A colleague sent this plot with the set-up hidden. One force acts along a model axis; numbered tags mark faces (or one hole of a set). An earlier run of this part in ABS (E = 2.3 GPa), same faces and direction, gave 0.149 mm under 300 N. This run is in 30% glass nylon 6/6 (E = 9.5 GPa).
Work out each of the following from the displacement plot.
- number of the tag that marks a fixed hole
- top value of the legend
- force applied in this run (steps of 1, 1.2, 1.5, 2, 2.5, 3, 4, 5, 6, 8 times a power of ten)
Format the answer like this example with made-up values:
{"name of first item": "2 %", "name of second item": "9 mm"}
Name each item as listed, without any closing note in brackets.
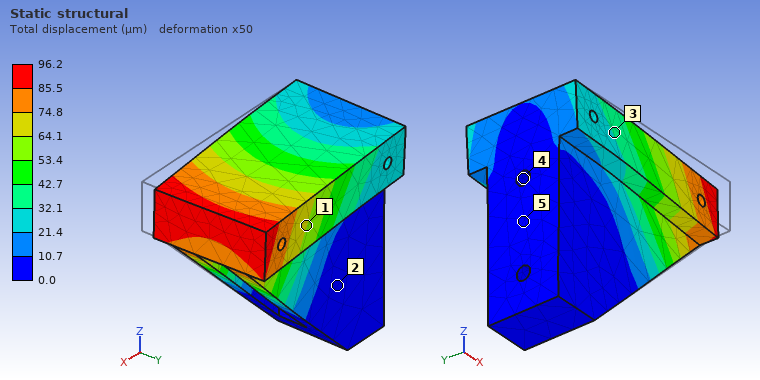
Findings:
{"number of the tag that marks a fixed hole": "4", "top value of the legend": "96.2 µm", "force applied in this run": "800 N"}
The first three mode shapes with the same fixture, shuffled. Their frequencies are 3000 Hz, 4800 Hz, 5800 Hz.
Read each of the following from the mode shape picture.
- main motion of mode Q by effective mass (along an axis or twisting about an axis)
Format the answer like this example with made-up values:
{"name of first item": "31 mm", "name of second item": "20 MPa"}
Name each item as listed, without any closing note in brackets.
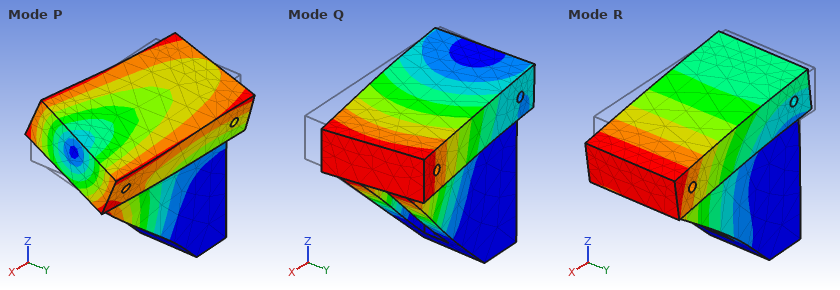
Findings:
{"main motion of mode Q by effective mass": "along Y"}
